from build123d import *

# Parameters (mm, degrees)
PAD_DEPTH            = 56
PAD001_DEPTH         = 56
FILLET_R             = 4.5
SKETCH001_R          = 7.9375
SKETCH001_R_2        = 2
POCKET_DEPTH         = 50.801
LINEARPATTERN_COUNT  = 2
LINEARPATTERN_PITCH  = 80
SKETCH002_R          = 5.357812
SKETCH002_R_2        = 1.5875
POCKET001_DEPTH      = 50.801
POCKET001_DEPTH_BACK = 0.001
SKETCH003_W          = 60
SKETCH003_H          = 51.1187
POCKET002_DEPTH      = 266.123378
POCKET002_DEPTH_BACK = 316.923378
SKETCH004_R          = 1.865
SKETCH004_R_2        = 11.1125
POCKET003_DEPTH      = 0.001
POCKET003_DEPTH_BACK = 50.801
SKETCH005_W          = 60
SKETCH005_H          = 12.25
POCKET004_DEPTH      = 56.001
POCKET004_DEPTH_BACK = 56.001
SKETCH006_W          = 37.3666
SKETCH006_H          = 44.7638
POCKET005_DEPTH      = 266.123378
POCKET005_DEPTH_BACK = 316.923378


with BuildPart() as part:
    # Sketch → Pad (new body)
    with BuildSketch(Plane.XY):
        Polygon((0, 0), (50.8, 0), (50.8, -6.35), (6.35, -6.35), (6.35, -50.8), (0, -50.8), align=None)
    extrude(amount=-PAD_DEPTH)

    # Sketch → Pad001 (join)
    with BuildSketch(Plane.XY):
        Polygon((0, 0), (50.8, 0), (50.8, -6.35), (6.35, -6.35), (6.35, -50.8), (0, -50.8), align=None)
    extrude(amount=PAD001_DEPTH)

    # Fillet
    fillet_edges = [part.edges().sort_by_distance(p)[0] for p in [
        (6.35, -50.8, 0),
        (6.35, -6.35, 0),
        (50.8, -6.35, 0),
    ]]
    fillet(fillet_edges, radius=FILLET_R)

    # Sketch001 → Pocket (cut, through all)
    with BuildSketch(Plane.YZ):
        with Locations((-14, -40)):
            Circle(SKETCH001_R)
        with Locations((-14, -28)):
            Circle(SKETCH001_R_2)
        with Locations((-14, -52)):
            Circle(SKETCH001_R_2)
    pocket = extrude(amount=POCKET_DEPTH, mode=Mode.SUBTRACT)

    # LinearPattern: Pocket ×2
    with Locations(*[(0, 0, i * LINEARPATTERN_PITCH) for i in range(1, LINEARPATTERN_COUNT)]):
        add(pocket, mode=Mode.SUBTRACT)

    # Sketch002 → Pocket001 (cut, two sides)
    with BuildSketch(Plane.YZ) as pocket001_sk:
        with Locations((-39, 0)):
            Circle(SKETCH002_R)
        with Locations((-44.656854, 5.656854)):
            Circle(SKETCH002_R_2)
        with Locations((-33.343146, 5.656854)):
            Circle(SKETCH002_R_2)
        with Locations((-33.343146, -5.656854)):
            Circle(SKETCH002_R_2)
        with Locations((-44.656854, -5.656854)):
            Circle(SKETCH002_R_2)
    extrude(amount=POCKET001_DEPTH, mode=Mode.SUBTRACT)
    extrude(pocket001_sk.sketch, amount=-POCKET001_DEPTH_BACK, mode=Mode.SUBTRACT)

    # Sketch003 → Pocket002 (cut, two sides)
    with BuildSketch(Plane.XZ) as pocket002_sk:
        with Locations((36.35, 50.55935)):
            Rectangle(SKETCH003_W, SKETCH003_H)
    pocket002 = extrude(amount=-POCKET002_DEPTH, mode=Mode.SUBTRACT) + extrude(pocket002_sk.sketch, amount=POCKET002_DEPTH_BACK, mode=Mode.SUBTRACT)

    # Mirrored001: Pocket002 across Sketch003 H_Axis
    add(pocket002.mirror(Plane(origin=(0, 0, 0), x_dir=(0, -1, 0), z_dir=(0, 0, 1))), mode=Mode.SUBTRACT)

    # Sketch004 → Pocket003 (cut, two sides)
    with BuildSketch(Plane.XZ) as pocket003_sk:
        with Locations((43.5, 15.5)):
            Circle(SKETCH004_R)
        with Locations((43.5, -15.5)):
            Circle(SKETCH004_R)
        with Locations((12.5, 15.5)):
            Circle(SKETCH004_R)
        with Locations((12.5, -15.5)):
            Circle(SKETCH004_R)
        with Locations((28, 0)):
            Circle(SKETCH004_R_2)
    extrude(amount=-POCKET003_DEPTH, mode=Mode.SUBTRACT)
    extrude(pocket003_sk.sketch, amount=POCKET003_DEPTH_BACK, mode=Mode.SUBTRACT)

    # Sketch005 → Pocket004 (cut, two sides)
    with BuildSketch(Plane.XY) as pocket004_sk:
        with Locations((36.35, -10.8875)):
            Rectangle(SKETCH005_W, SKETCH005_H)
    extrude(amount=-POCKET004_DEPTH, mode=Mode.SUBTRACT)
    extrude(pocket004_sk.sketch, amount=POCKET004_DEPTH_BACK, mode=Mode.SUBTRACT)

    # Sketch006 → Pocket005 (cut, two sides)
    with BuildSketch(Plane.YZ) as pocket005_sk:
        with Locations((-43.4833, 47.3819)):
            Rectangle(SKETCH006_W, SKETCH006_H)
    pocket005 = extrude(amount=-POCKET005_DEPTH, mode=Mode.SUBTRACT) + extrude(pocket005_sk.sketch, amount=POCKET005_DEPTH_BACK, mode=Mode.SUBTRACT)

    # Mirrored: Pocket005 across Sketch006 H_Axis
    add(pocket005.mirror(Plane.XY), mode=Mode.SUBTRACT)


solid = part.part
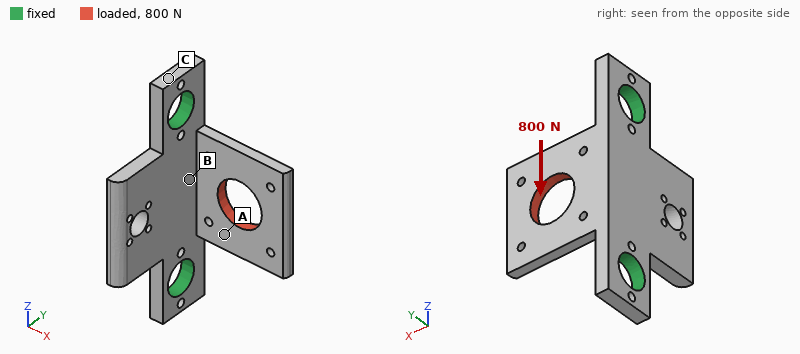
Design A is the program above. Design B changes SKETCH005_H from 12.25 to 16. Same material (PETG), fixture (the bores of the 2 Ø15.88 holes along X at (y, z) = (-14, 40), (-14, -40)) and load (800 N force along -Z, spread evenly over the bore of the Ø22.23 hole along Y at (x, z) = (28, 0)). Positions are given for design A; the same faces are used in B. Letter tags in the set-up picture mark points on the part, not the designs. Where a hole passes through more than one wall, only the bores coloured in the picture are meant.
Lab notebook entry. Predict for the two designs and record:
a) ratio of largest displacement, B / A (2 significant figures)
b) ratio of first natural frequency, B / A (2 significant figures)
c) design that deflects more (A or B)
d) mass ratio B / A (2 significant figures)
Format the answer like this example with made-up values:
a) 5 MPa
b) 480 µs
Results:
a) 1.5
b) 0.70
c) B
d) 0.89
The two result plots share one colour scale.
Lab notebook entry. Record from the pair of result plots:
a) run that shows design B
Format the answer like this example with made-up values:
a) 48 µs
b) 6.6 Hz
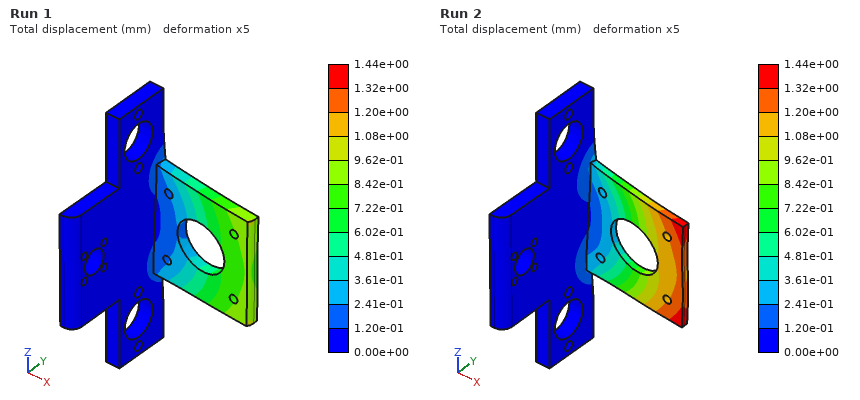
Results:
a) Run 2
